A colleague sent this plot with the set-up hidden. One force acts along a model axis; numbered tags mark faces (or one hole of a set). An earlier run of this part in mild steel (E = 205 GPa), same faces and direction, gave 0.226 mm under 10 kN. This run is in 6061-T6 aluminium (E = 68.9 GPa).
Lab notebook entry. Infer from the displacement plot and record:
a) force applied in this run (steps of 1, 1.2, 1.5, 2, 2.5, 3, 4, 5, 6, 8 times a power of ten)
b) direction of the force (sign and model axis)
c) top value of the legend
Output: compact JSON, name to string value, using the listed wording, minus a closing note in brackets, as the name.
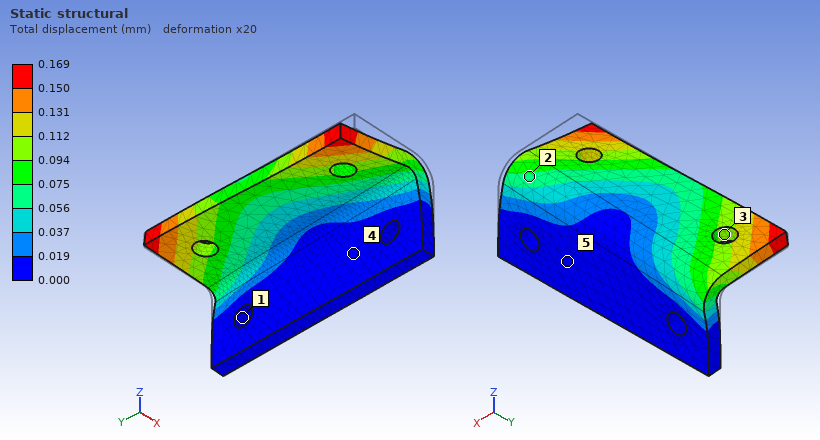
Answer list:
{"force applied in this run": "2.5 kN", "direction of the force": "+Y", "top value of the legend": "0.169 mm"}
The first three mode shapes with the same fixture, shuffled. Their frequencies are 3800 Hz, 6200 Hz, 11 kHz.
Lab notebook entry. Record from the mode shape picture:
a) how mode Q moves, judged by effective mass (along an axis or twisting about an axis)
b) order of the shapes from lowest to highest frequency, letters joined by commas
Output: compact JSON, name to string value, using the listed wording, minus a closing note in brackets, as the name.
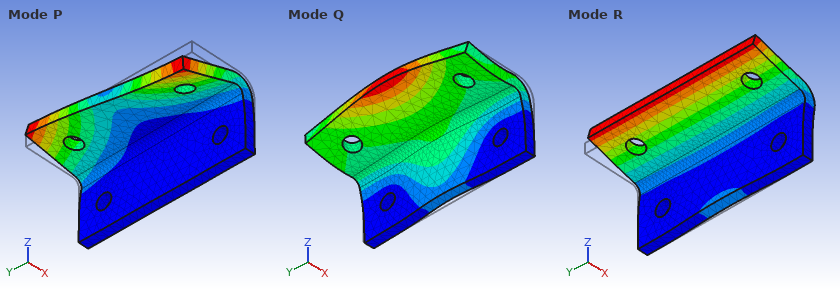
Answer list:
{"how mode Q moves, judged by effective mass": "along X", "order of the shapes from lowest to highest frequency, letters joined by commas": "R, P, Q"}
